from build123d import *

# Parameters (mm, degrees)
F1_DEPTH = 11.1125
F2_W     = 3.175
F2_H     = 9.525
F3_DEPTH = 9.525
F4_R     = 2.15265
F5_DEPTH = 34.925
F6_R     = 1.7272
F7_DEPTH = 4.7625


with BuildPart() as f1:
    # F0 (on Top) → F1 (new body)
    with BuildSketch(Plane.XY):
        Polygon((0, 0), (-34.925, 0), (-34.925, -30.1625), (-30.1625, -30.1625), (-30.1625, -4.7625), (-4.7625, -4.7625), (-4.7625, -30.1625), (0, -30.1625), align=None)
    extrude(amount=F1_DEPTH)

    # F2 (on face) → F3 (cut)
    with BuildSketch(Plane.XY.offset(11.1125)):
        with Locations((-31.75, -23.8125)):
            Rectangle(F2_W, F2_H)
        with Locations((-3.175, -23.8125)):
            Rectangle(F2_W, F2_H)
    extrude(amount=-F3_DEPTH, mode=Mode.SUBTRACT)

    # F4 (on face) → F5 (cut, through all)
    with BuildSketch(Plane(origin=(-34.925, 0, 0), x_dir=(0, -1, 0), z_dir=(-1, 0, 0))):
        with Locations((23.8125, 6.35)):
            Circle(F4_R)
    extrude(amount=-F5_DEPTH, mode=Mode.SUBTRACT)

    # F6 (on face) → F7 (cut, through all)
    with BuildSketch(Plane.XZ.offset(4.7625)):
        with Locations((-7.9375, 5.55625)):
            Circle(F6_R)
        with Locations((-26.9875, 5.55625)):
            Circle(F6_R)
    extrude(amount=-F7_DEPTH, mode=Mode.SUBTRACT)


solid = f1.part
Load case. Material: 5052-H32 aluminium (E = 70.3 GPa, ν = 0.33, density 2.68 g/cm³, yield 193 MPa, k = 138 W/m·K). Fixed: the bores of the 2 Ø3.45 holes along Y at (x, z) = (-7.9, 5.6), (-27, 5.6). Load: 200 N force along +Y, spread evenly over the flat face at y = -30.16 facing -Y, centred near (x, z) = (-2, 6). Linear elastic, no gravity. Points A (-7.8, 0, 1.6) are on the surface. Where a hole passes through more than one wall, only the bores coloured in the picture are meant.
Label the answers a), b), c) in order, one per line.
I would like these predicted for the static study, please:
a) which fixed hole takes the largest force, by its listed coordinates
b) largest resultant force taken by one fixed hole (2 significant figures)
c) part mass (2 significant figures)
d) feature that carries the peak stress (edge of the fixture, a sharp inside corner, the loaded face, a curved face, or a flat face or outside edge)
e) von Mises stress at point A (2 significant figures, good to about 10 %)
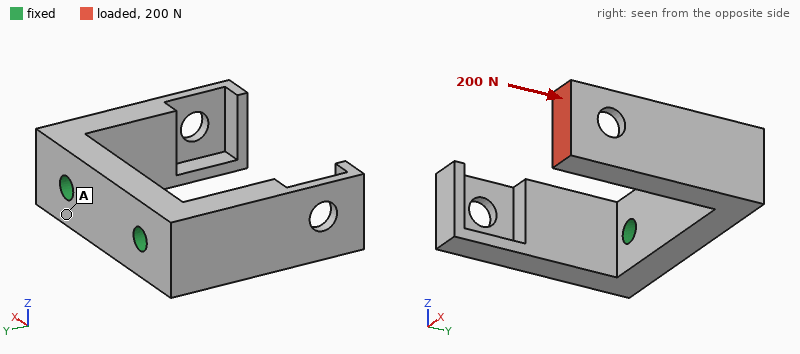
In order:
a) (-7.9, 5.6)
b) 210 N
c) 10 g
d) a curved face
e) 8.6 MPa
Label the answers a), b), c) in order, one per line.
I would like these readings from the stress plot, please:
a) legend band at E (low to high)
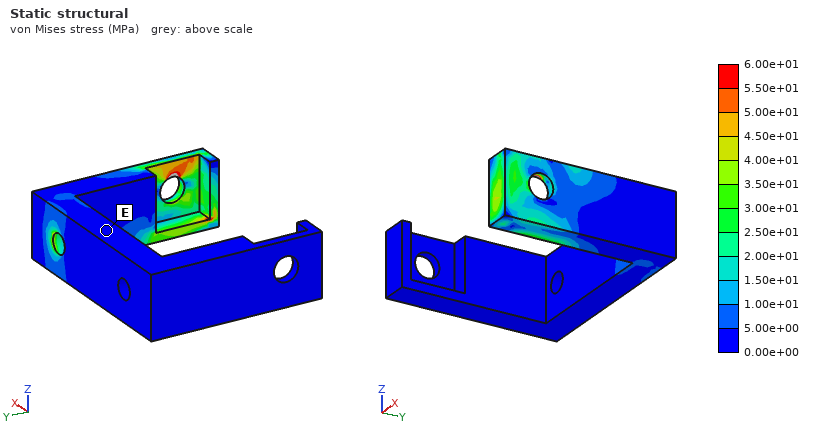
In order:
a) 0.00e+00 to 5.00e+00 MPa
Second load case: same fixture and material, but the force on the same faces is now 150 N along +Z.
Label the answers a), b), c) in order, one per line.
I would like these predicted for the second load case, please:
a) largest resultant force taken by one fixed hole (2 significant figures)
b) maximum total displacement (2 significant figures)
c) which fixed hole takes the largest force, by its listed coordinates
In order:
a) 170 N
b) 0.11 mm
c) (-7.9, 5.6)
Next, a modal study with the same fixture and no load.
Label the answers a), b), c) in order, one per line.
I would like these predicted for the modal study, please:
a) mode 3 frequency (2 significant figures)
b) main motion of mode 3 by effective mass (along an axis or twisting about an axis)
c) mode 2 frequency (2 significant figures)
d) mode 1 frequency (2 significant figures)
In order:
a) 7700 Hz
b) along Z
c) 5000 Hz
d) 5000 Hz
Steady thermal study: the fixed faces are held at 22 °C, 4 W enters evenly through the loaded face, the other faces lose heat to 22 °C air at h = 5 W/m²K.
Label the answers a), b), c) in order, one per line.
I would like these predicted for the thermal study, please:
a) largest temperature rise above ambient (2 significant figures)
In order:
a) 31 K
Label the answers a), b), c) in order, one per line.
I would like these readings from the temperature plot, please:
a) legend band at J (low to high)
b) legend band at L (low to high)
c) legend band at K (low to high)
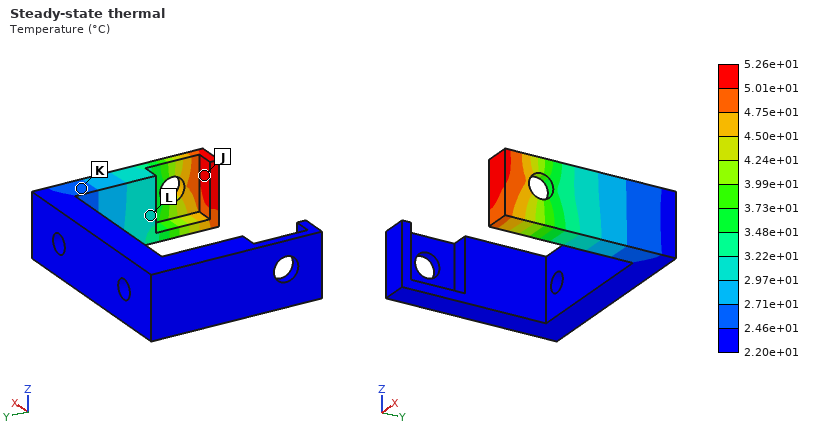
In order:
a) 5.01e+01 to 5.26e+01 °C
b) 2.97e+01 to 3.22e+01 °C
c) 2.46e+01 to 2.71e+01 °C
